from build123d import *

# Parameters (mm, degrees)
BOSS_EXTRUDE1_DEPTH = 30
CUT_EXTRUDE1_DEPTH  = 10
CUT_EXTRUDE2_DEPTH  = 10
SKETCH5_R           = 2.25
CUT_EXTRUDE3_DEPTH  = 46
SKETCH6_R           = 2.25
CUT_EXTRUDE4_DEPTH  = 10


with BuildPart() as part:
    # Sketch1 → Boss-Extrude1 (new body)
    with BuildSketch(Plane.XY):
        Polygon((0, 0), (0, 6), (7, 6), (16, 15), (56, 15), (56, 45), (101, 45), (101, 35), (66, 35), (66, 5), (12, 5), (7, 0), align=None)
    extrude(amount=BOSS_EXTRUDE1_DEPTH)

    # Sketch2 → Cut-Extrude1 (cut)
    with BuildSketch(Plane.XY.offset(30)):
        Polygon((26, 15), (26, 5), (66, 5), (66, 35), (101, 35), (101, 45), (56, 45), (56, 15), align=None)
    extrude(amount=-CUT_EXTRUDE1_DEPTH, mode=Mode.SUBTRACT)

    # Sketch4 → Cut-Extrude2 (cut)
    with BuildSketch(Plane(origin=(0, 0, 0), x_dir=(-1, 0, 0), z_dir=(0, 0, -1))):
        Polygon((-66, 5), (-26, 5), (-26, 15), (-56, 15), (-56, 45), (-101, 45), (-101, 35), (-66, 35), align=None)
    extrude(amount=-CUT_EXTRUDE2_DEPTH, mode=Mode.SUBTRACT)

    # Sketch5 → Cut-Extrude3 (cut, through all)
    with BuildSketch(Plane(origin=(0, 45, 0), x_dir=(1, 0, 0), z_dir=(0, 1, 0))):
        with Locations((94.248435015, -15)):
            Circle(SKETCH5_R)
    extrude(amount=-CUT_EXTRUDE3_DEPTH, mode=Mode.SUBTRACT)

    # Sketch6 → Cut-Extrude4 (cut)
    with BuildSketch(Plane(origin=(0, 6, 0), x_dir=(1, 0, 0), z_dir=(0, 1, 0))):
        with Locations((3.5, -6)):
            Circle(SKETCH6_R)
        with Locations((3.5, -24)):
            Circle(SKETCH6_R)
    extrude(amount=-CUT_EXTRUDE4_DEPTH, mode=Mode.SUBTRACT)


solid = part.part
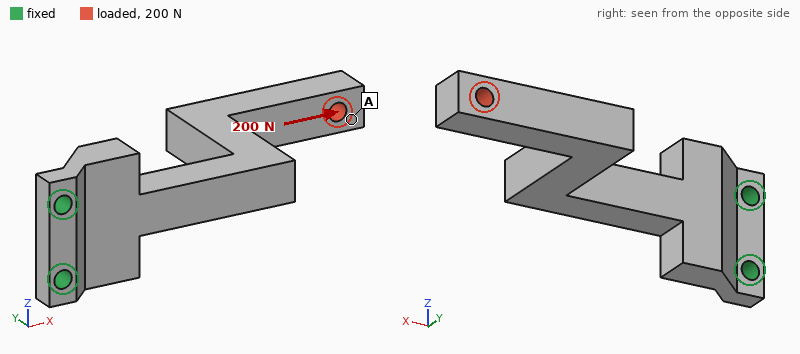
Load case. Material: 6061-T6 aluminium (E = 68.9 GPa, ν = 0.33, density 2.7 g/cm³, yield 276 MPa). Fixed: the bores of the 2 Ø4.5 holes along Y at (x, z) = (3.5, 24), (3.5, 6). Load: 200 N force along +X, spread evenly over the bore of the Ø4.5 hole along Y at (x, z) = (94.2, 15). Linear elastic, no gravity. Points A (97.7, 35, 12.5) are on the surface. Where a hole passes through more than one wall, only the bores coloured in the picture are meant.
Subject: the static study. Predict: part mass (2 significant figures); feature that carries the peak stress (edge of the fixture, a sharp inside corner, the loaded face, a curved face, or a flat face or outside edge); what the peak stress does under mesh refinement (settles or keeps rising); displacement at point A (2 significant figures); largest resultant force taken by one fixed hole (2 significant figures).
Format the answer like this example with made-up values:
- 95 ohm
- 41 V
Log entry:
- 44 g
- a sharp inside corner
- keeps rising
- 0.70 mm
- 100 N
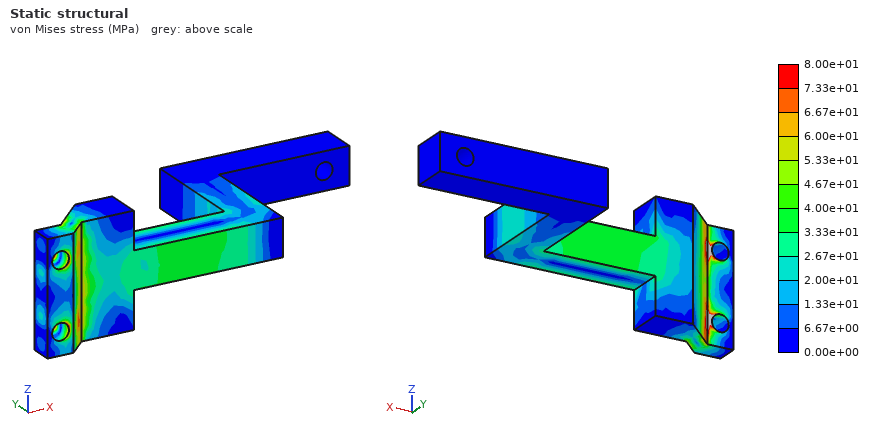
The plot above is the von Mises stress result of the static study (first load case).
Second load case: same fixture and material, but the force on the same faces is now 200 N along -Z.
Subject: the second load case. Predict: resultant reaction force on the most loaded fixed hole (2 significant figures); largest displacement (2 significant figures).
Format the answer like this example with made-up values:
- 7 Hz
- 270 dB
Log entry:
- 950 N
- 0.90 mm
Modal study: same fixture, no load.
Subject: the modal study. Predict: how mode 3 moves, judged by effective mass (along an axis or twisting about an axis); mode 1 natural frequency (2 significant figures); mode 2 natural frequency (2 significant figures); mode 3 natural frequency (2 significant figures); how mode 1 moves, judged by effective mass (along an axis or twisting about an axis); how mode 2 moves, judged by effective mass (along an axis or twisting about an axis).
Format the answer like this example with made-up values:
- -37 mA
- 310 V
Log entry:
- along Y
- 530 Hz
- 900 Hz
- 2600 Hz
- along Y
- along Z
